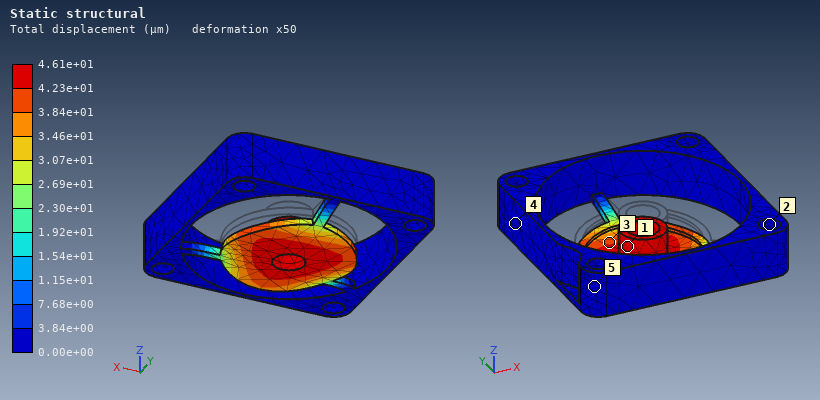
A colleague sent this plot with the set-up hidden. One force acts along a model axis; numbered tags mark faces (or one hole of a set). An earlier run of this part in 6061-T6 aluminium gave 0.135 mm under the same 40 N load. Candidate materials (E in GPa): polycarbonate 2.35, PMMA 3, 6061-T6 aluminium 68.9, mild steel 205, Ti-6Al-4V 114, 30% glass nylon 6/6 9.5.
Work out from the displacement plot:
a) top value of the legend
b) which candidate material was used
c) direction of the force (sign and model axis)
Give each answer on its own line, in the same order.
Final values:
4.61e+01 µm
mild steel
-Z
